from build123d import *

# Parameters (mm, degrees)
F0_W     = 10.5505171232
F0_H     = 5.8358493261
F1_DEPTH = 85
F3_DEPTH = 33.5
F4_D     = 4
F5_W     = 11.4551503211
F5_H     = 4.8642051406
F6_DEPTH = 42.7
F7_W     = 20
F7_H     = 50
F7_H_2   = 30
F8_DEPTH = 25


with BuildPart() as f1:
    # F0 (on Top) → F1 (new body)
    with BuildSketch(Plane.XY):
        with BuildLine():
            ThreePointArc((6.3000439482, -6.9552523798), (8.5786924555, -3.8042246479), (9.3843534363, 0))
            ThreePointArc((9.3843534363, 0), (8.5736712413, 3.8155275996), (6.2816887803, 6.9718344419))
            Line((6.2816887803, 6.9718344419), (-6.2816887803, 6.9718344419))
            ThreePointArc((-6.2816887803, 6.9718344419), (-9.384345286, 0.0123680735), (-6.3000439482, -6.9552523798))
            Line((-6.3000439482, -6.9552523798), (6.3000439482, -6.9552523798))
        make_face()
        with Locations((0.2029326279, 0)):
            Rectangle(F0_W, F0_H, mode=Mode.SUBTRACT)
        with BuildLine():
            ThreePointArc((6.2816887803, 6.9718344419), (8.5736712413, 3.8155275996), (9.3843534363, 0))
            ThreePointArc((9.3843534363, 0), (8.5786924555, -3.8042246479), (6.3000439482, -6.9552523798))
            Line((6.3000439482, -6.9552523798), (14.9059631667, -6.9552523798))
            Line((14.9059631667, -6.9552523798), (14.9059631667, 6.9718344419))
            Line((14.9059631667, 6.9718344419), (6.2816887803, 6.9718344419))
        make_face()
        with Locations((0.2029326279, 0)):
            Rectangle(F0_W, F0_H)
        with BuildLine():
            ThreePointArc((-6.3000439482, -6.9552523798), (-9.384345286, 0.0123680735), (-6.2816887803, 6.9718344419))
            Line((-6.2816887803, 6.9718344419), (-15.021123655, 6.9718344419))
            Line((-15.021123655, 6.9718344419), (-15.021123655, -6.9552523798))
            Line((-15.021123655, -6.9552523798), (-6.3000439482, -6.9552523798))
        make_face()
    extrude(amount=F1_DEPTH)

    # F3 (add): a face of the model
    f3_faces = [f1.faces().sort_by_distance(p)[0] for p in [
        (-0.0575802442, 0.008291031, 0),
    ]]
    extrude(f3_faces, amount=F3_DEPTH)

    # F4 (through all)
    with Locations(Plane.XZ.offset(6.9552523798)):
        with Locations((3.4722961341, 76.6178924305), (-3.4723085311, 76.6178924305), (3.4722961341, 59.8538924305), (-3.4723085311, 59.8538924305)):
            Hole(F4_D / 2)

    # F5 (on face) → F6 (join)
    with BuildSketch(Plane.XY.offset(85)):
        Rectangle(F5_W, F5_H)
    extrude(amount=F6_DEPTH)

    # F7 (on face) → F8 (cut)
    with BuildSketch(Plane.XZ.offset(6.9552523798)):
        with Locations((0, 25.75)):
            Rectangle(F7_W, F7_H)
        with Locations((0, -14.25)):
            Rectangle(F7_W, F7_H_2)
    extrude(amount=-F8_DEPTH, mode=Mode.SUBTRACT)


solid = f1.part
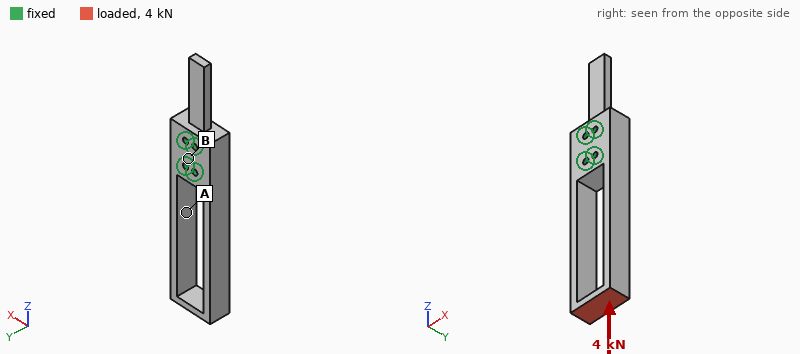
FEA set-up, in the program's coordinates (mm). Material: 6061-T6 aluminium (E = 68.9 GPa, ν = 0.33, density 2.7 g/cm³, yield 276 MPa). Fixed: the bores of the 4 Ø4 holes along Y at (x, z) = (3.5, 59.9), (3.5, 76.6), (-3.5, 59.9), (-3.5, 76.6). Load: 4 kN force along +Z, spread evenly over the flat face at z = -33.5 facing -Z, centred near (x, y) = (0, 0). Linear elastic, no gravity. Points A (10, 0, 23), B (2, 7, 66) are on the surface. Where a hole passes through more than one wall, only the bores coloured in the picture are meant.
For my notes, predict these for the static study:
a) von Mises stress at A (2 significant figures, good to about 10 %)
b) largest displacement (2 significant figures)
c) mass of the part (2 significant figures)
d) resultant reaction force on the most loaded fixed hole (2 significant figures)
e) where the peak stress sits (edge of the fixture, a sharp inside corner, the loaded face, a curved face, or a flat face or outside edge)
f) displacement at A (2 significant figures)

34 MPa
0.11 mm
78 g
1.2 kN
a flat face or outside edge
0.067 mm
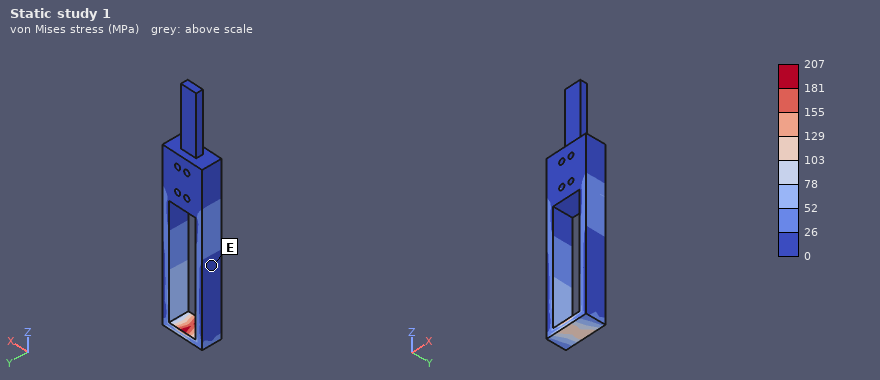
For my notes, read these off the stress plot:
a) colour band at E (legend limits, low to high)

0 to 26 MPa
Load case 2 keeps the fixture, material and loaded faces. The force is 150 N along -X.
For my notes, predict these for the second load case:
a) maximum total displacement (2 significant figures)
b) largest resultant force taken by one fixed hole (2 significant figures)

0.46 mm
420 N
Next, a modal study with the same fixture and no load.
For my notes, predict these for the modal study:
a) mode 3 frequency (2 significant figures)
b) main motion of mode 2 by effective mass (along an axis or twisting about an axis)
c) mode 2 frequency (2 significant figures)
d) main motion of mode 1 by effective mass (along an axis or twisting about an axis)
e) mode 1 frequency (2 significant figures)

2000 Hz
along Y
1100 Hz
along X
740 Hz
